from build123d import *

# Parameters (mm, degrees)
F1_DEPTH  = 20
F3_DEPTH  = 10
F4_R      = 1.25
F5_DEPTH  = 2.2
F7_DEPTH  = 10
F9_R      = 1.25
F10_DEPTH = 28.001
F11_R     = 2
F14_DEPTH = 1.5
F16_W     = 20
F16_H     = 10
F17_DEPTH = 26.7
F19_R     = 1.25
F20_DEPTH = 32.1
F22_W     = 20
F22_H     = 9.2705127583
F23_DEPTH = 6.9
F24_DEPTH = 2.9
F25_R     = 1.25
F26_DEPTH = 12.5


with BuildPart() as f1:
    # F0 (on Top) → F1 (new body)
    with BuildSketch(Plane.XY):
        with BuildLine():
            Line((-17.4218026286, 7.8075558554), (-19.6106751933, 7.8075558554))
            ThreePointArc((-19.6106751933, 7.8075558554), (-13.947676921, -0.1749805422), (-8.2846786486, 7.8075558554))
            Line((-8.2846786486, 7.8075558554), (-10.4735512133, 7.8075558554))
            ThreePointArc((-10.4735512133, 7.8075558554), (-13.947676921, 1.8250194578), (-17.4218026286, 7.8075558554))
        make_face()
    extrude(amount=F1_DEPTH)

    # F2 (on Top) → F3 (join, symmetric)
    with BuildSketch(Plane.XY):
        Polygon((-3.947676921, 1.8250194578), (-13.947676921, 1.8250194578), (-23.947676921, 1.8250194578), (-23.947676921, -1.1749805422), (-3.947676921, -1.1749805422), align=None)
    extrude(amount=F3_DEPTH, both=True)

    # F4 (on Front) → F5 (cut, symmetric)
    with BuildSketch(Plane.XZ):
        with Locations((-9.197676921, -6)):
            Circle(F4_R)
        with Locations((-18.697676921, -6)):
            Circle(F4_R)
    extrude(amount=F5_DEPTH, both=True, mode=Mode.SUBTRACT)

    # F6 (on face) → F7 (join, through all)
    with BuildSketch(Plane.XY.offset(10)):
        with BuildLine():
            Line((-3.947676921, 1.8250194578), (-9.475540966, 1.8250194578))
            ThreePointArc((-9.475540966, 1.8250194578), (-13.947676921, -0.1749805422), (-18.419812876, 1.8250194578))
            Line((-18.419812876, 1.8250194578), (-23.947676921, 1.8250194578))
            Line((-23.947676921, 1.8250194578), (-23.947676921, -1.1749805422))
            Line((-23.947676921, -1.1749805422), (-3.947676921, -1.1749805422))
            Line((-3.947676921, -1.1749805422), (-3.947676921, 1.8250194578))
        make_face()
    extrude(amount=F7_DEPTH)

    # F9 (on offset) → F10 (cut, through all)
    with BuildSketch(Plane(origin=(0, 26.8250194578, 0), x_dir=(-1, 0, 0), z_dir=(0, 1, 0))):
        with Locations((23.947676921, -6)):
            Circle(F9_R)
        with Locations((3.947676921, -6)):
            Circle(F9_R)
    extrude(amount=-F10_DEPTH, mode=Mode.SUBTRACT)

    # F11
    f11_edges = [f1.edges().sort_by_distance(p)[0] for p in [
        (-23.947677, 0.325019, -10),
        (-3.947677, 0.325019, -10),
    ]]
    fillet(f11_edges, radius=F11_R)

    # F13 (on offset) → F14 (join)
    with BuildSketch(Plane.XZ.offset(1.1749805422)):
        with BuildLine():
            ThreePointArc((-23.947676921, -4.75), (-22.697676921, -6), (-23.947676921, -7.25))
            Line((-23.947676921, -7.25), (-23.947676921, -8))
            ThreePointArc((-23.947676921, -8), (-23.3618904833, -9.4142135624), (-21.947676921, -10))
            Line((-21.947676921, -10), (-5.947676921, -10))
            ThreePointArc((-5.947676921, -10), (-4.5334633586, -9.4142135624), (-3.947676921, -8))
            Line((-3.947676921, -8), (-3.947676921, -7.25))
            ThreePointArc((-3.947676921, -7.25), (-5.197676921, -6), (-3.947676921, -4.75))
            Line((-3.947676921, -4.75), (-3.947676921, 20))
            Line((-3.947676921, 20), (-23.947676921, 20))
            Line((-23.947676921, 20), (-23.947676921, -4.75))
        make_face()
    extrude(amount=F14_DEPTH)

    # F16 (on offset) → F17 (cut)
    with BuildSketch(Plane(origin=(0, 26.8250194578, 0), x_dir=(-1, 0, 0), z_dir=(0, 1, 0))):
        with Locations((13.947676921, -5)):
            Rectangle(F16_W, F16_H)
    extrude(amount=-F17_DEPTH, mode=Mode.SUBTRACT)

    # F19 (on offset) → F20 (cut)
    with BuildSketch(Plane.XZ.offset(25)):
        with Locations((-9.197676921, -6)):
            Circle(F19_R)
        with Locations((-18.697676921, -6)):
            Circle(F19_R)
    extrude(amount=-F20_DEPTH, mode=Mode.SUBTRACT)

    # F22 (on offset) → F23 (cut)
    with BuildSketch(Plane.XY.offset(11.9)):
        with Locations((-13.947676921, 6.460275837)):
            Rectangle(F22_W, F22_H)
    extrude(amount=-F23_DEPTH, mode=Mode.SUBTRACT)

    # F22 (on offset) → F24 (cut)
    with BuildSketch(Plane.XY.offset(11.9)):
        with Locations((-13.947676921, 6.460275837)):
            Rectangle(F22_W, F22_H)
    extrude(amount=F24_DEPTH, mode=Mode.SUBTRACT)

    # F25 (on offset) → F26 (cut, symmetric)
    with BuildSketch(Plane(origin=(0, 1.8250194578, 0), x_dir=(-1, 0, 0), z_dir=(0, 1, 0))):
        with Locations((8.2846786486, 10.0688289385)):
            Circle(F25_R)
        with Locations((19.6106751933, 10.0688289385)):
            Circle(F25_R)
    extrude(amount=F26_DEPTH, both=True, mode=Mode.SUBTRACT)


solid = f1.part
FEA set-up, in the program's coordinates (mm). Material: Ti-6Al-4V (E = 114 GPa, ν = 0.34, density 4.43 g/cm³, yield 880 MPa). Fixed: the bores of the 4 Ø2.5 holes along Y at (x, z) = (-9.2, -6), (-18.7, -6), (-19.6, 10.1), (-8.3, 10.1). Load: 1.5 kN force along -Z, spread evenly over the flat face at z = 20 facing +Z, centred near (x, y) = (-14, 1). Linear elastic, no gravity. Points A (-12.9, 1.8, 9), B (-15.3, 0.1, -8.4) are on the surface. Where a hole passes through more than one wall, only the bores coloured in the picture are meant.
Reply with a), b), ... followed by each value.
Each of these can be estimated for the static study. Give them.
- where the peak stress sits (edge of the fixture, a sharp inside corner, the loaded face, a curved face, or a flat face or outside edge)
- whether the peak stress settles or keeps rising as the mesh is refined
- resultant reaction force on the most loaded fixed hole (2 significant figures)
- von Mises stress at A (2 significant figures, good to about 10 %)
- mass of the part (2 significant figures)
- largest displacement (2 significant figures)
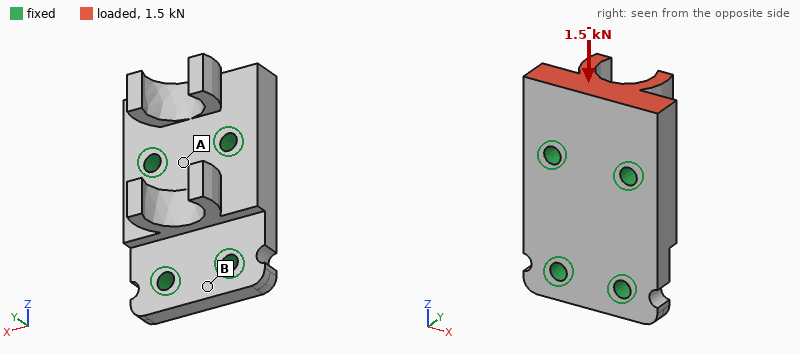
a) edge of the fixture
b) keeps rising
c) 710 N
d) 17 MPa
e) 11 g
f) 14 µm
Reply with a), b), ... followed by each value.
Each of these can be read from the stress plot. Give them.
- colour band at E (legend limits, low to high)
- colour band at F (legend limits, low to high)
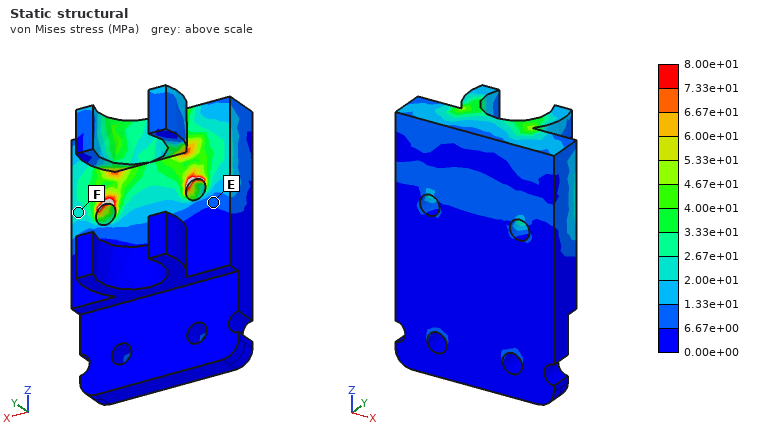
a) 6.67e+00 to 1.33e+01 MPa
b) 2.00e+01 to 2.67e+01 MPa
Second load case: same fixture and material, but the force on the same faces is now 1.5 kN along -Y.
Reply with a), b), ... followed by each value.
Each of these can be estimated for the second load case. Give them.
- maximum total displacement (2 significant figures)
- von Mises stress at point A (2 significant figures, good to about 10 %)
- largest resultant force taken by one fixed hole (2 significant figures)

a) 52 µm
b) 73 MPa
c) 830 N
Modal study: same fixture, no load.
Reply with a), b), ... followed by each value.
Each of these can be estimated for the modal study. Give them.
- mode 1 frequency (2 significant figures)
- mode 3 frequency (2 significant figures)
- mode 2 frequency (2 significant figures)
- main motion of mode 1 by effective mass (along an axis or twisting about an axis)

a) 26 kHz
b) 35 kHz
c) 31 kHz
d) along Y
